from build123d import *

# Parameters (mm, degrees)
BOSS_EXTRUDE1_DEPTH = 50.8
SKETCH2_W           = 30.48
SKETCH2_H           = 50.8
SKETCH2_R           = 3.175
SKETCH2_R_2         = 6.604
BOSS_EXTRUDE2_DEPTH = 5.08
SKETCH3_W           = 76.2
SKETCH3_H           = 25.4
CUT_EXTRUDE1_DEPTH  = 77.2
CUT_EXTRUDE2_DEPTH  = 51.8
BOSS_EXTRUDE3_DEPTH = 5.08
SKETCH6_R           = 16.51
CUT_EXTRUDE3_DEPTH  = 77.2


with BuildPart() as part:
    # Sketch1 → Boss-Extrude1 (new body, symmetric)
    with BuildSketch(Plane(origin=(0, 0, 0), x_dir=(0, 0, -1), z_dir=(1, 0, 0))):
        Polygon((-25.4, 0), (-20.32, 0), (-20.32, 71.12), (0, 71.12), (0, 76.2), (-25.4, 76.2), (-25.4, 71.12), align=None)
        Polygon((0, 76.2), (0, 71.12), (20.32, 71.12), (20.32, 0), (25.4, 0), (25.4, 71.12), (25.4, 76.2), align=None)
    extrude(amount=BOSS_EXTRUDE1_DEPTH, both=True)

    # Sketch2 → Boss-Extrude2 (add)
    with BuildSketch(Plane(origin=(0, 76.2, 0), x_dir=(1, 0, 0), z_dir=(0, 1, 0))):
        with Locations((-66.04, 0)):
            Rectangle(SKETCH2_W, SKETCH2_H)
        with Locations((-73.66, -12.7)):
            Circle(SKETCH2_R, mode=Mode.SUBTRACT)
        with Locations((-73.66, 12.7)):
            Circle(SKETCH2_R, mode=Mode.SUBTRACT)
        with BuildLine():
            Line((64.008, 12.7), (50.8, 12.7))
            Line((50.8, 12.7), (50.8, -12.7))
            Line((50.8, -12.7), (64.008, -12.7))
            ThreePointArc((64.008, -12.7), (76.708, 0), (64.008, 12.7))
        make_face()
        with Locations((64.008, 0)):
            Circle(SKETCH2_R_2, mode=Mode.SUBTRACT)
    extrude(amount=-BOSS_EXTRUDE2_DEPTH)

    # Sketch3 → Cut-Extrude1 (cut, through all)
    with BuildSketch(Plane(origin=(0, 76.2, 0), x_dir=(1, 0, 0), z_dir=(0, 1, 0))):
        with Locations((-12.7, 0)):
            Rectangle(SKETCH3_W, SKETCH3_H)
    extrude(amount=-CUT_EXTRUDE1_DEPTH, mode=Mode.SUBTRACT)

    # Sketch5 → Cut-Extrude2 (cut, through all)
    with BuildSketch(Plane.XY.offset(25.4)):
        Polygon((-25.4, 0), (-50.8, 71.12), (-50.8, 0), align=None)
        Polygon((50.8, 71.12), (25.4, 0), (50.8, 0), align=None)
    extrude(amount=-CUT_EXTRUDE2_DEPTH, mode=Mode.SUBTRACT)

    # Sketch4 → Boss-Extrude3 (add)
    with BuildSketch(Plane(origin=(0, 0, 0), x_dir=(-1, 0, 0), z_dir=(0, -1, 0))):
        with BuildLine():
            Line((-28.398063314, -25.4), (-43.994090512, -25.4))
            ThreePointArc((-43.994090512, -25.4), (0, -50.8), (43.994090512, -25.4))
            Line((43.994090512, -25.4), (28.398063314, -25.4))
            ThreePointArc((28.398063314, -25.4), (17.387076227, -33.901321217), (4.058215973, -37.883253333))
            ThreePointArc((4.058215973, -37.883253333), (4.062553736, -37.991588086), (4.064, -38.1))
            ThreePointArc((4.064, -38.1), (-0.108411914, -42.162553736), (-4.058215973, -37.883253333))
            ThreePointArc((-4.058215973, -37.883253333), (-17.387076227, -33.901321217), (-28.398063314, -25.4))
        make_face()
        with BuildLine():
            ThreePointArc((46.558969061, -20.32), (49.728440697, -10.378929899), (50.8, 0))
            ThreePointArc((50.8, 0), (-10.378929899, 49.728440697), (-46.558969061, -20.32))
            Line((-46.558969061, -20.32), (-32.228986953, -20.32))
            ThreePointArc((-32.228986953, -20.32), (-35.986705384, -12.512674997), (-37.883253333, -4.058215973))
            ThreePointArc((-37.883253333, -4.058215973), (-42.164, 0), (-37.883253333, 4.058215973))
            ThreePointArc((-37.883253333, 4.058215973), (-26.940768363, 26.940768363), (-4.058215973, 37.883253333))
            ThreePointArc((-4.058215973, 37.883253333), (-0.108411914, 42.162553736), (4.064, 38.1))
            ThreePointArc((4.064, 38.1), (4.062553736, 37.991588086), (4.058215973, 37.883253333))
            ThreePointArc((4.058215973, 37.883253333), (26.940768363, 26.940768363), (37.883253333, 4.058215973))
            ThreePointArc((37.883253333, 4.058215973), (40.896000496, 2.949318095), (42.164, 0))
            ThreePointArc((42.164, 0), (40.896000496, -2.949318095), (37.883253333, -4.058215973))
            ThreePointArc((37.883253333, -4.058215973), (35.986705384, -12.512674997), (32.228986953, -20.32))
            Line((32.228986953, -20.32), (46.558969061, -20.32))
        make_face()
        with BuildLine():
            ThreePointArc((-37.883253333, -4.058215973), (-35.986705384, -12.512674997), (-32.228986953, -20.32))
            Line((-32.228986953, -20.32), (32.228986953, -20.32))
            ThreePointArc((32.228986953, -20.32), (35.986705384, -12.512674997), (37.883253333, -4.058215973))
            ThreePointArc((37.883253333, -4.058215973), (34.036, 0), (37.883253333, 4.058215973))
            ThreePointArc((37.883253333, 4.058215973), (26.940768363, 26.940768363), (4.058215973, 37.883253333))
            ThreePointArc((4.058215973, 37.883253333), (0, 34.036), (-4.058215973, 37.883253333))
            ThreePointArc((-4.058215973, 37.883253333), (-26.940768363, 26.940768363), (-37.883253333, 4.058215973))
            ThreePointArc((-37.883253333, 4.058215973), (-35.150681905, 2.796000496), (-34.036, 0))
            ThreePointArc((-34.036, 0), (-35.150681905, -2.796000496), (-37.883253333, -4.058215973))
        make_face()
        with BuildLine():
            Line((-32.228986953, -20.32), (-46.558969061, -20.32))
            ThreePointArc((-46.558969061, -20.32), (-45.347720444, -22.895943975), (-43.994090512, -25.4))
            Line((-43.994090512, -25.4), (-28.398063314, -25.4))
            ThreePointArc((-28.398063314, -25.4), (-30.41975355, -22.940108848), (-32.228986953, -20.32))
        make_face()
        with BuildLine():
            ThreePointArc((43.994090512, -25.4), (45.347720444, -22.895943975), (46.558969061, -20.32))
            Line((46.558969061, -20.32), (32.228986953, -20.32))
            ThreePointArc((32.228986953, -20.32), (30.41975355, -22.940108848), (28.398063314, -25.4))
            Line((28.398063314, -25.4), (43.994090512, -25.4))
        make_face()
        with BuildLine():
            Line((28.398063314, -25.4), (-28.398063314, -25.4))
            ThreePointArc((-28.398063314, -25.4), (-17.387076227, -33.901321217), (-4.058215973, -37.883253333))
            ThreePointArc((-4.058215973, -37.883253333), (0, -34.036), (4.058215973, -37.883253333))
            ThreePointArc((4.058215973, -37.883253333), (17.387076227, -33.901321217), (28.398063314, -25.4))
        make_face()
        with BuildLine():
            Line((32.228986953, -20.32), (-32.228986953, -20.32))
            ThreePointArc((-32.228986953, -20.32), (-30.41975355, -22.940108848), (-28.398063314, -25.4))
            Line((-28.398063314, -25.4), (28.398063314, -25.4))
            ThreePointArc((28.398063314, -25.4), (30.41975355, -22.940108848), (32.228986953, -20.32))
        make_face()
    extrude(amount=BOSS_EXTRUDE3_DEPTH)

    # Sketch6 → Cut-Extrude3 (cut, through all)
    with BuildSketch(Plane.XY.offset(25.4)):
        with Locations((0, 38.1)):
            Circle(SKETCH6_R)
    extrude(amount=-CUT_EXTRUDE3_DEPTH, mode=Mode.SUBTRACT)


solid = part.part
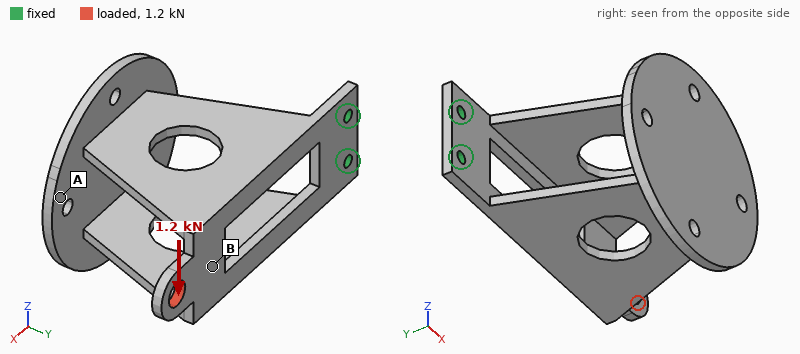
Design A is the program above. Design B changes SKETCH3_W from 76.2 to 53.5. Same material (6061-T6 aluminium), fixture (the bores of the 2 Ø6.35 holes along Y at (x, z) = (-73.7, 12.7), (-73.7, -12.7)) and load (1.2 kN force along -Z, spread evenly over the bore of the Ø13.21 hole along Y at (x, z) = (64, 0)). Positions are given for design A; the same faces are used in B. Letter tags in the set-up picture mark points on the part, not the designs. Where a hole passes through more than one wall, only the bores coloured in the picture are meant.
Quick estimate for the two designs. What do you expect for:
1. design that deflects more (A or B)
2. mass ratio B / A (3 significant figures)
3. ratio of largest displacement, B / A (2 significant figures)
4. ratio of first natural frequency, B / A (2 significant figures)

A
1.03
0.64
1.1
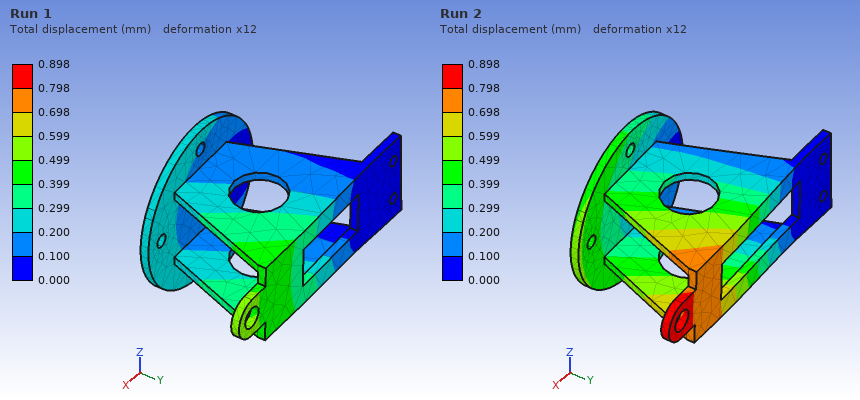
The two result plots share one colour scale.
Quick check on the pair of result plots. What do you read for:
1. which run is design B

Run 1
